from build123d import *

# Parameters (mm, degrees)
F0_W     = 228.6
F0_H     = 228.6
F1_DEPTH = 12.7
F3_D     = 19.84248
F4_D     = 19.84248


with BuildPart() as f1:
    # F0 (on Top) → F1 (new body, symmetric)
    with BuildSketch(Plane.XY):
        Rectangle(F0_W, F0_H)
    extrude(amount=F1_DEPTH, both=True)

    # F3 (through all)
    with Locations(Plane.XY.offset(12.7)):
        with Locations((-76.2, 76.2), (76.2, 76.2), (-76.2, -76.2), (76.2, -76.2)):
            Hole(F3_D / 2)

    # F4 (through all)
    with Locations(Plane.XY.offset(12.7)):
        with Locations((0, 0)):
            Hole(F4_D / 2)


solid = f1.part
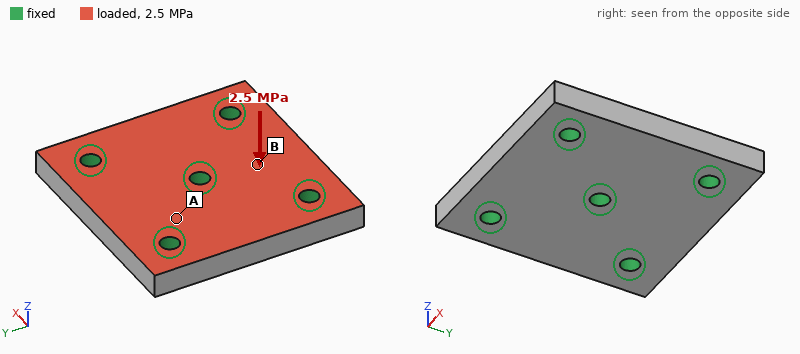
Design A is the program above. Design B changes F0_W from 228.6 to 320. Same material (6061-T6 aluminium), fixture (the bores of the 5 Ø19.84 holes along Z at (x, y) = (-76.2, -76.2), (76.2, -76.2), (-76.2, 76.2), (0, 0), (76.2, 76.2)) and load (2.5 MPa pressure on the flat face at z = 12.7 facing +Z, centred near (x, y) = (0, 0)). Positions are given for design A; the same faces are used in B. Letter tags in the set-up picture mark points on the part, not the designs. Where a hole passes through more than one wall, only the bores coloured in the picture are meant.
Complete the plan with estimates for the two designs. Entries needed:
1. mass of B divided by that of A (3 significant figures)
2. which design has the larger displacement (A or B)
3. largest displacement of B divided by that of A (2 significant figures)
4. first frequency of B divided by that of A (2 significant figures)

1.41
B
5.3
0.47
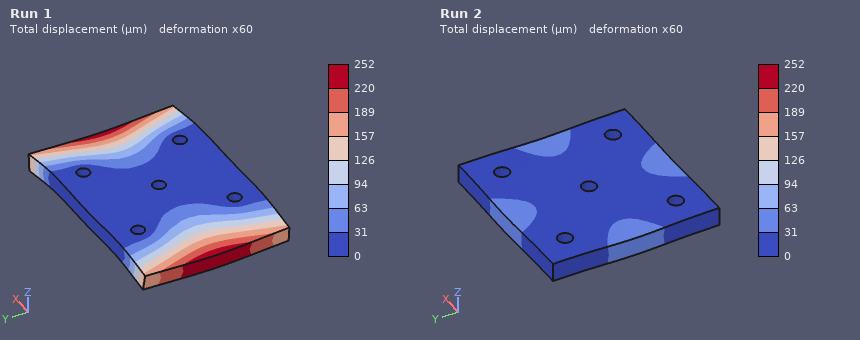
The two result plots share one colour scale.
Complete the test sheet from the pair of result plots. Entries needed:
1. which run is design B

Run 1
